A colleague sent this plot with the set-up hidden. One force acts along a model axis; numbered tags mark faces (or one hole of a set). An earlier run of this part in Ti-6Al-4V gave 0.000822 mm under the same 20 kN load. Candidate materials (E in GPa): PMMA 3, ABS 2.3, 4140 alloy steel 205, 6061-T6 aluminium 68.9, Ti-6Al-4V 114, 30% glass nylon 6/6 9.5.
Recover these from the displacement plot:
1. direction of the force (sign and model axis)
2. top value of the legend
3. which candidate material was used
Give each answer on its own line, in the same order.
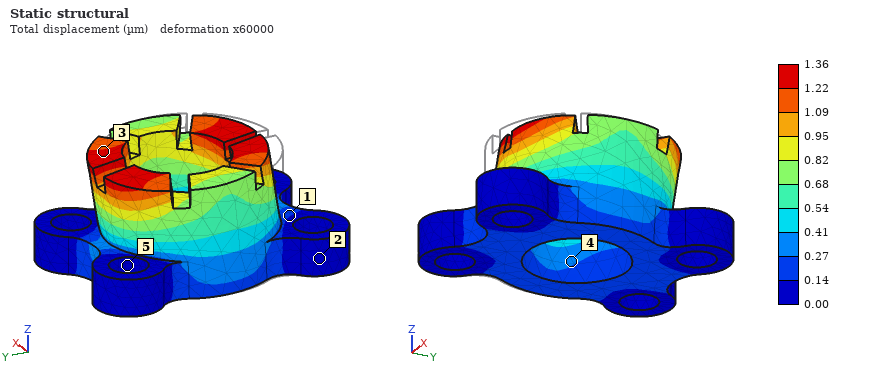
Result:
+Y
1.36 µm
6061-T6 aluminium
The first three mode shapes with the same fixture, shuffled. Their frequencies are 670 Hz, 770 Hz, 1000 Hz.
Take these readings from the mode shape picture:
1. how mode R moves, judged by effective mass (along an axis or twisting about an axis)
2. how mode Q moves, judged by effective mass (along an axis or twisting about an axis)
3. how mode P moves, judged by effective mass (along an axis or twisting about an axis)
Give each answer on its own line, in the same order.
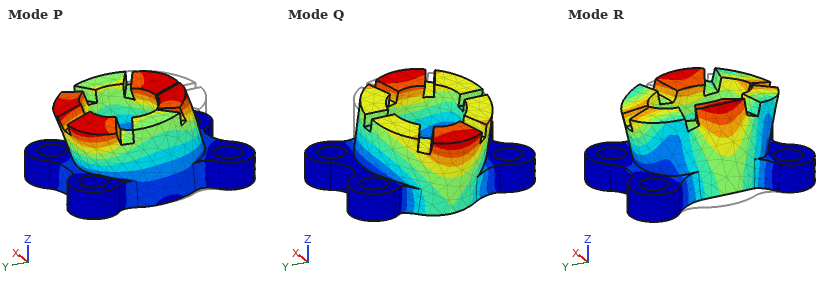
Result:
along Z
along X
along Y
